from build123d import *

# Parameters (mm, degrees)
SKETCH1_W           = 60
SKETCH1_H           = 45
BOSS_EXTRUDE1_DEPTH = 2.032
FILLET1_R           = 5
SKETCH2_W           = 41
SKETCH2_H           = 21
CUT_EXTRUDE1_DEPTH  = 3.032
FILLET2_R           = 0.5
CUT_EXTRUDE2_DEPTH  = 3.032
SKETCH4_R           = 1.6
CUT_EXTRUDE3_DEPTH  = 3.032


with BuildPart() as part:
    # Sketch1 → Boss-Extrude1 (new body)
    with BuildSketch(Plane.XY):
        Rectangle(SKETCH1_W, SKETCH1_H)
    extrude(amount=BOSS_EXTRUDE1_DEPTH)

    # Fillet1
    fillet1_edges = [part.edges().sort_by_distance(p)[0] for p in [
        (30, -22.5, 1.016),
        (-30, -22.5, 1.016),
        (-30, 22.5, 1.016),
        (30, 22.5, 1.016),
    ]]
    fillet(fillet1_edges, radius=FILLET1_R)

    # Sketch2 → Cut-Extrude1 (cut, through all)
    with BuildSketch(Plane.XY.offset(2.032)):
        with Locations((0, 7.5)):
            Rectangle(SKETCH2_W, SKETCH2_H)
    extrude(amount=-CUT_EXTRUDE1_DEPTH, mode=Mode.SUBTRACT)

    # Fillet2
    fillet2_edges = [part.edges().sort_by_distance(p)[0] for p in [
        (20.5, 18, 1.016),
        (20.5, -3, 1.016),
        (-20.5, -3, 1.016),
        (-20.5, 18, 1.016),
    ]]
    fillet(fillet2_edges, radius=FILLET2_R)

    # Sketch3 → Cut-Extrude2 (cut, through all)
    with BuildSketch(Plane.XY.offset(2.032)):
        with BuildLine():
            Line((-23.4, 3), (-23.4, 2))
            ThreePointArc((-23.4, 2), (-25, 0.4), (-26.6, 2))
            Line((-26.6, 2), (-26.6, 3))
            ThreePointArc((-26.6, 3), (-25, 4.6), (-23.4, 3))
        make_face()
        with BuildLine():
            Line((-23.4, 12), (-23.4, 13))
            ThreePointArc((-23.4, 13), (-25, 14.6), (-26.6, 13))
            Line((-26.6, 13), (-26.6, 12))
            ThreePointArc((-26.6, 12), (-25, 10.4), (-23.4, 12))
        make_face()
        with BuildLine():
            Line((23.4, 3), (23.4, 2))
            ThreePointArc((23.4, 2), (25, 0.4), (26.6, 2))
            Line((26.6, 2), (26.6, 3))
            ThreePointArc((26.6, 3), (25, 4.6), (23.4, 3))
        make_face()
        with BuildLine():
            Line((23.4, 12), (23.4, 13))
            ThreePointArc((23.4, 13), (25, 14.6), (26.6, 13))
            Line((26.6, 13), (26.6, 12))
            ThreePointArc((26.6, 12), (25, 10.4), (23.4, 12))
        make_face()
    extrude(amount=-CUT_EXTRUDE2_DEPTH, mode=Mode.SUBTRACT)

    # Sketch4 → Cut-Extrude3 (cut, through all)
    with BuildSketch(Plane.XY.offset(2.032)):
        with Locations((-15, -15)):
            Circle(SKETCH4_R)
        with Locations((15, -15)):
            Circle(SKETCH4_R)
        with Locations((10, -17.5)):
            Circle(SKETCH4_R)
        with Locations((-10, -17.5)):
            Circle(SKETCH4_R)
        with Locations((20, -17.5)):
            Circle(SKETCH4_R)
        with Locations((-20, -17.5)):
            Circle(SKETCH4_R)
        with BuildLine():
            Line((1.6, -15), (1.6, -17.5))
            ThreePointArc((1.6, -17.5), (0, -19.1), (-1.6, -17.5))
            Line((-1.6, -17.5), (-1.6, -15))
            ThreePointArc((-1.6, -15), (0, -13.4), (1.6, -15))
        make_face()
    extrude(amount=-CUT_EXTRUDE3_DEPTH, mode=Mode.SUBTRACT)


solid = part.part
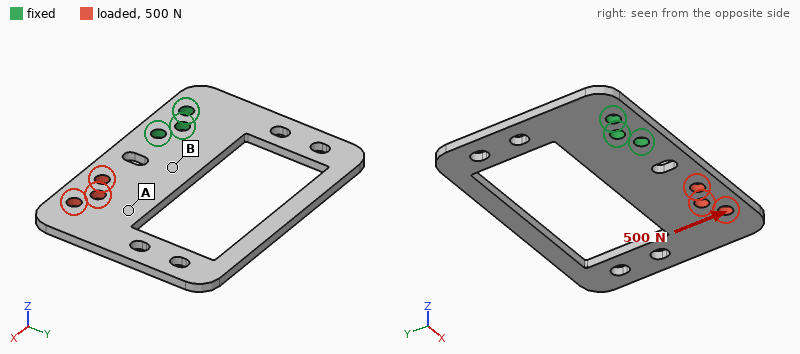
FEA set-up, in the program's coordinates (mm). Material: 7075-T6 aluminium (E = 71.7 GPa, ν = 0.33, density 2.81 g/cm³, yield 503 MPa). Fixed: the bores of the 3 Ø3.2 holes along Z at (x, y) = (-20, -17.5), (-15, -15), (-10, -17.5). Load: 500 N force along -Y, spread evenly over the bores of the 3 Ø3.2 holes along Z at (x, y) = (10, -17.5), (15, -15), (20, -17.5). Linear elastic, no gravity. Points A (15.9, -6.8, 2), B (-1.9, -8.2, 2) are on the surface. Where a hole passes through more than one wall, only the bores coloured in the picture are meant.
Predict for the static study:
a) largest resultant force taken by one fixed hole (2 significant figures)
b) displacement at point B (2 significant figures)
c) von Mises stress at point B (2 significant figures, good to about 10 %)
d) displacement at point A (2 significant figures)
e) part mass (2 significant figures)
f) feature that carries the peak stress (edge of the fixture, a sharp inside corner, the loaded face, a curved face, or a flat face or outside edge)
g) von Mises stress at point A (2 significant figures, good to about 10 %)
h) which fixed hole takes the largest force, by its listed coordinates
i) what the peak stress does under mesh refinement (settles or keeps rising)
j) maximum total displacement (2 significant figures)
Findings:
1.3 kN
0.026 mm
39 MPa
0.082 mm
9.8 g
edge of the fixture
13 MPa
(-10, -17.5)
keeps rising
0.13 mm
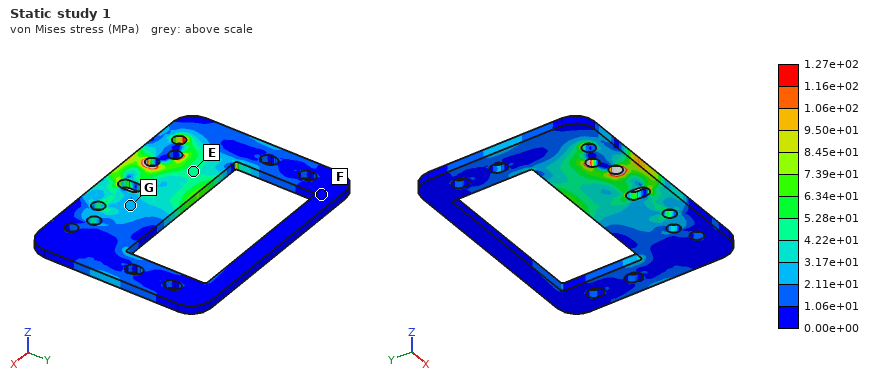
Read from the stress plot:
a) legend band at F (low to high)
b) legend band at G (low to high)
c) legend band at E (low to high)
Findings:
0.00e+00 to 1.06e+01 MPa
2.11e+01 to 3.17e+01 MPa
4.22e+01 to 5.28e+01 MPa
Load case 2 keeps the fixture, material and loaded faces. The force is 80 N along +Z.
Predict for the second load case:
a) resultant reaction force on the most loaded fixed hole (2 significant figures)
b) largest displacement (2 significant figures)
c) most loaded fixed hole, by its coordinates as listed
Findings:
180 N
0.87 mm
(-10, -17.5)
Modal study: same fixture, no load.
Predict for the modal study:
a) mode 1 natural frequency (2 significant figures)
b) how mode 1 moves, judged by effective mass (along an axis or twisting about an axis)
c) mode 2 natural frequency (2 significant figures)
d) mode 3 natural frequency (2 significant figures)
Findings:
610 Hz
along Z
1100 Hz
1800 Hz
